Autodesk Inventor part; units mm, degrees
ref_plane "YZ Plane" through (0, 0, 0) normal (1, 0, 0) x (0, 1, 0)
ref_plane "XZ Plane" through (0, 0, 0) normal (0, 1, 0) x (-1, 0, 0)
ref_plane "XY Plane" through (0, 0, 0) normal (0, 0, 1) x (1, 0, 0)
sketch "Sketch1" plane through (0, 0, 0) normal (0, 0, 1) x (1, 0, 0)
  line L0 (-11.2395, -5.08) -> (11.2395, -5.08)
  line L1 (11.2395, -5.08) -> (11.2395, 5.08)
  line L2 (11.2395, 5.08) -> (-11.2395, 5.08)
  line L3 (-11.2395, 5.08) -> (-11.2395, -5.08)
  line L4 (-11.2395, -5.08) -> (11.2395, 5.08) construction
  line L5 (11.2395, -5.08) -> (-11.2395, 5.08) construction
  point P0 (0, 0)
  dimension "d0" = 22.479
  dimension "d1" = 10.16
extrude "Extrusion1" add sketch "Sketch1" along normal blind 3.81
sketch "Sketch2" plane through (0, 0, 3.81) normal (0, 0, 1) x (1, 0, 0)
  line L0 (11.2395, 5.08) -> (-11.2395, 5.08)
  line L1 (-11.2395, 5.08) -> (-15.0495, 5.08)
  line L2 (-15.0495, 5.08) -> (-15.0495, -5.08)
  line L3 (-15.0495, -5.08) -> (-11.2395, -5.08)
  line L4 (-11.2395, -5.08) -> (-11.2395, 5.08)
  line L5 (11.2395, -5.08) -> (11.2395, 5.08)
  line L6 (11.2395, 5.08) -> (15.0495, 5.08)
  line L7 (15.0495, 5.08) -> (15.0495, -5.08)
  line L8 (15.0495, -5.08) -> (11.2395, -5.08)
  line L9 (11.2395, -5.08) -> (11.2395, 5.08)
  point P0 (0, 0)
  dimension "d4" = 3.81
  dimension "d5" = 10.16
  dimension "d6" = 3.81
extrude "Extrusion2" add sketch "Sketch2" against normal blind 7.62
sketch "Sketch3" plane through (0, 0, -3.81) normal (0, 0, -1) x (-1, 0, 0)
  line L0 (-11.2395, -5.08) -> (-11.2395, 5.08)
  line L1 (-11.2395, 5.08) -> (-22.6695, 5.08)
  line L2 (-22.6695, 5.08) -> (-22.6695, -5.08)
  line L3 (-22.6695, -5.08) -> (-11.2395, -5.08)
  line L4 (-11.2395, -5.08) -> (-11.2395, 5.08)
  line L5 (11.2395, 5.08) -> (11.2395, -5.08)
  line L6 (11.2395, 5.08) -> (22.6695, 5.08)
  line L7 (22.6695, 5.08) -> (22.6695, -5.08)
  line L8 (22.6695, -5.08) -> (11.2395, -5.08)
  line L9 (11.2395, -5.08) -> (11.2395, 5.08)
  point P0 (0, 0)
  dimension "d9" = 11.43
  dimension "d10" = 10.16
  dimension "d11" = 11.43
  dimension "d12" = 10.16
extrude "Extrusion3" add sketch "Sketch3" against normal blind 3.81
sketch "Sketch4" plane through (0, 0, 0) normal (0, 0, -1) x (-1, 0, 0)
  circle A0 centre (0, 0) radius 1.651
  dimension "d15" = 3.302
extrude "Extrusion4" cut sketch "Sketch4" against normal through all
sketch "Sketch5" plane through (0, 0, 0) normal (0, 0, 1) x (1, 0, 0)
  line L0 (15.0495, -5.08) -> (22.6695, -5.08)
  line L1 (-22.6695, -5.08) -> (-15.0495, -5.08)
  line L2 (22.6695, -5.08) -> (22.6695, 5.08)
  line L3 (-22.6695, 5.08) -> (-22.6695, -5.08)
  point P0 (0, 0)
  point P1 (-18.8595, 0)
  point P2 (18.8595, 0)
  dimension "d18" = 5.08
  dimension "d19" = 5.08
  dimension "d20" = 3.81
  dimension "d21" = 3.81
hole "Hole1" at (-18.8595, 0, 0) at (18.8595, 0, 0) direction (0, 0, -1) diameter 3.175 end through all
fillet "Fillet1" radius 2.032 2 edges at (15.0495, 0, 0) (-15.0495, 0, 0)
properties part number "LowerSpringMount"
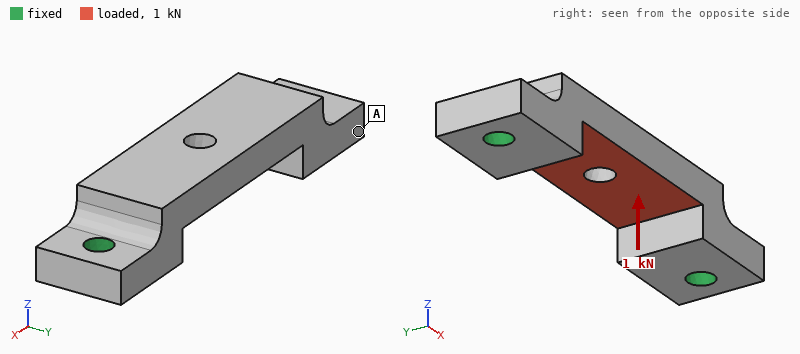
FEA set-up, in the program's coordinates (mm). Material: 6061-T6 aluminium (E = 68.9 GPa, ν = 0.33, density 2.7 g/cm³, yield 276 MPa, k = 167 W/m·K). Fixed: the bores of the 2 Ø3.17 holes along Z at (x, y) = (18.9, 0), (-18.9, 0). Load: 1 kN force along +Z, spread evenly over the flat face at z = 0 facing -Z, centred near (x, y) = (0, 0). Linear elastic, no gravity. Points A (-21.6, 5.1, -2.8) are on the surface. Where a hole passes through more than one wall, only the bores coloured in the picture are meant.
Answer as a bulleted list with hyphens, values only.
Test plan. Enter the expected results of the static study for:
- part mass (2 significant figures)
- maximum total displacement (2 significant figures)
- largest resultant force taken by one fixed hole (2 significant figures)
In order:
- 5.3 g
- 39 µm
- 920 N
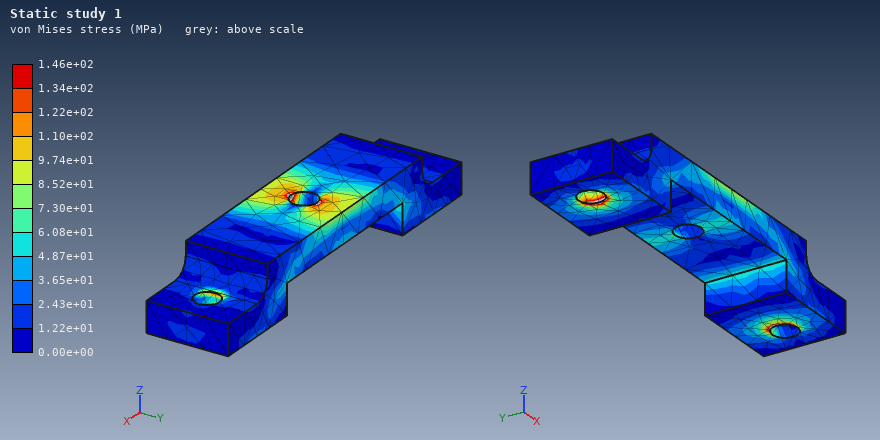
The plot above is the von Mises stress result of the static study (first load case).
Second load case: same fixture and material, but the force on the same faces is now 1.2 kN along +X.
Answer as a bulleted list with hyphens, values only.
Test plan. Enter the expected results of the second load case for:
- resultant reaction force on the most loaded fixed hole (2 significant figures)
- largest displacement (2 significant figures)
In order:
- 600 N
- 11 µm
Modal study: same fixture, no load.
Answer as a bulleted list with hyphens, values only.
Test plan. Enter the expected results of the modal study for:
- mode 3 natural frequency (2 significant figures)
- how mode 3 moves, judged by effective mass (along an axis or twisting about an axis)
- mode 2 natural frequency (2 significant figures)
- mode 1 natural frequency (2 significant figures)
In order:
- 28 kHz
- along X
- 19 kHz
- 19 kHz
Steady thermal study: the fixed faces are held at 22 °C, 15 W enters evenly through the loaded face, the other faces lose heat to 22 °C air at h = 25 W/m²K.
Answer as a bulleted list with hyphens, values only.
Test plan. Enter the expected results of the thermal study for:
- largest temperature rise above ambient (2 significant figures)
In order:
- 15 K
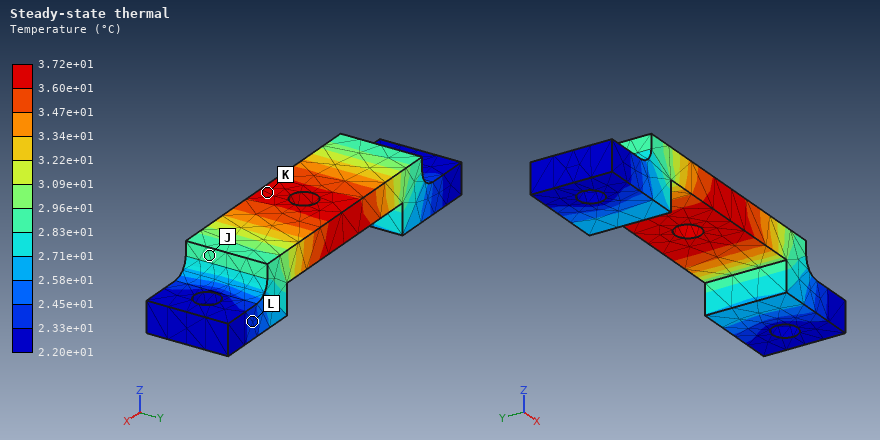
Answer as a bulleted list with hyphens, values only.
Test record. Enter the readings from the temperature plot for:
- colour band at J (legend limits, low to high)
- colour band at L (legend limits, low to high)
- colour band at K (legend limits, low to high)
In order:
- 2.83e+01 to 2.96e+01 °C
- 2.33e+01 to 2.45e+01 °C
- 3.60e+01 to 3.72e+01 °C
